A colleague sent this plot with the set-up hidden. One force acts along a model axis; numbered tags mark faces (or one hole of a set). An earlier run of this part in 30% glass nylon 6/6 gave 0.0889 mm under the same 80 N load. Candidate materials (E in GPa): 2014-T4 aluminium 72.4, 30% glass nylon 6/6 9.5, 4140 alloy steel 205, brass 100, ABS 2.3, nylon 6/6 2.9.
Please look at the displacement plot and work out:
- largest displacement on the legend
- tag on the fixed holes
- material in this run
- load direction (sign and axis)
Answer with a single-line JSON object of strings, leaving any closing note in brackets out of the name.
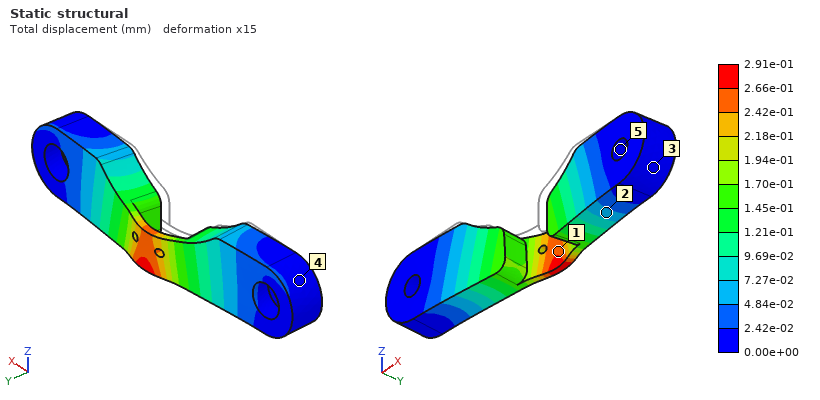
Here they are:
{"largest displacement on the legend": "2.91e-01 mm", "tag on the fixed holes": "5", "material in this run": "nylon 6/6", "load direction": "+Y"}
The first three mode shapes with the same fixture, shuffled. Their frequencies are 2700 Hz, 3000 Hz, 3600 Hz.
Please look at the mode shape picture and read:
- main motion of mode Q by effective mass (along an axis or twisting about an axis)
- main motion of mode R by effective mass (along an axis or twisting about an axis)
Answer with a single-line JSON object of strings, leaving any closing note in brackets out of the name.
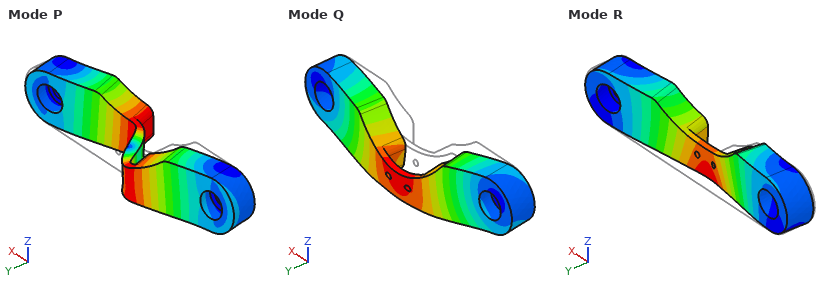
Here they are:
{"main motion of mode Q by effective mass": "along Z", "main motion of mode R by effective mass": "along Y"}
